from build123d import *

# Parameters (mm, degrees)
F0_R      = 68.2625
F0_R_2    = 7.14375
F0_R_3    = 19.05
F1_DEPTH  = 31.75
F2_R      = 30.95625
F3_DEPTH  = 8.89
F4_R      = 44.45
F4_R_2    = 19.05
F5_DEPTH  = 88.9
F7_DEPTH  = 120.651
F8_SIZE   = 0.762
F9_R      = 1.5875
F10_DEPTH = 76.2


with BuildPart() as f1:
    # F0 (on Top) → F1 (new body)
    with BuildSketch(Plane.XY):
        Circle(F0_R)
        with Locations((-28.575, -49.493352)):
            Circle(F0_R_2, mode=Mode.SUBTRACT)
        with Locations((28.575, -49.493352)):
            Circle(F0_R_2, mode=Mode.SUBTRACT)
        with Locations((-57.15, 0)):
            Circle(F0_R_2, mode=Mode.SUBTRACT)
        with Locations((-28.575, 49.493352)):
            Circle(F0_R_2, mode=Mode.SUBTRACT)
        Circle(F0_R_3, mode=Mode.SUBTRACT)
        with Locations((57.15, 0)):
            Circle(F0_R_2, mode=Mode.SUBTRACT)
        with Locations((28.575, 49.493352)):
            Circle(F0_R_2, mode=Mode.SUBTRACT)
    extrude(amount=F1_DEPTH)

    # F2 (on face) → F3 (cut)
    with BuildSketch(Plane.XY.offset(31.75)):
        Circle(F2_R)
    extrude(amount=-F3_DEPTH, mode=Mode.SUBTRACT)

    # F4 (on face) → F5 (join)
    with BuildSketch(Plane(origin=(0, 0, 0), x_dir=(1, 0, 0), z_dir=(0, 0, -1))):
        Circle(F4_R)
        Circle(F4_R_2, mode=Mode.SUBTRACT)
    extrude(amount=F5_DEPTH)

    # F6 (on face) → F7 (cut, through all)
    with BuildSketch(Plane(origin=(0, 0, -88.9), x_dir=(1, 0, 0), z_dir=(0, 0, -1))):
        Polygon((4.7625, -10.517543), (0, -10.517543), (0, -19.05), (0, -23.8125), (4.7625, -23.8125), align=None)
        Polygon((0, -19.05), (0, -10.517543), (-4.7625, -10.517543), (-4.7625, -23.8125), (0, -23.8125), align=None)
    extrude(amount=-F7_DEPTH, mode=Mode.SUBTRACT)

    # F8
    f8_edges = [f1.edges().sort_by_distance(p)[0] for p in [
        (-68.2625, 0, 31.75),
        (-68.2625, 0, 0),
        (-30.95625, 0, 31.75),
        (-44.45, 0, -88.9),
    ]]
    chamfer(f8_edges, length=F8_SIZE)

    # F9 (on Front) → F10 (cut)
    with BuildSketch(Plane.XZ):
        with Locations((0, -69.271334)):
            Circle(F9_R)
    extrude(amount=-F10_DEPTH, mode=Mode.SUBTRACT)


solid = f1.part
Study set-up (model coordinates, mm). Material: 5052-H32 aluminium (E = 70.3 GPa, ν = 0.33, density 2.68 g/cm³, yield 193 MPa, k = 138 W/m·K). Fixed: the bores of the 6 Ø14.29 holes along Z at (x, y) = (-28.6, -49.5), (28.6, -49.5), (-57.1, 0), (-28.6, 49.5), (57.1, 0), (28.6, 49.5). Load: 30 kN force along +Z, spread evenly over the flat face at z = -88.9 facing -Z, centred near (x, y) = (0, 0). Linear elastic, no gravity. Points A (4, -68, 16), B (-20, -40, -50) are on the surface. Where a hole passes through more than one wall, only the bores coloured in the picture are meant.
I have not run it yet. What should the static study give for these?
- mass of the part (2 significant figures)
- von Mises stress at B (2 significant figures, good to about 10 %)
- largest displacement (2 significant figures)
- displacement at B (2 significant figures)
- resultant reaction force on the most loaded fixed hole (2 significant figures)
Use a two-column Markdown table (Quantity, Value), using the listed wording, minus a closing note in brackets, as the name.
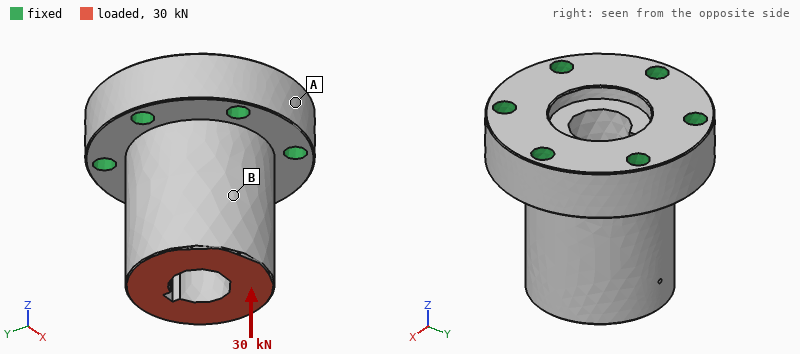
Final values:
| Quantity | Value |
|---|---|
| mass of the part | 2.2 kg |
| von Mises stress at B | 5.5 MPa |
| largest displacement | 11 µm |
| displacement at B | 7.9 µm |
| resultant reaction force on the most loaded fixed hole | 5.5 kN |
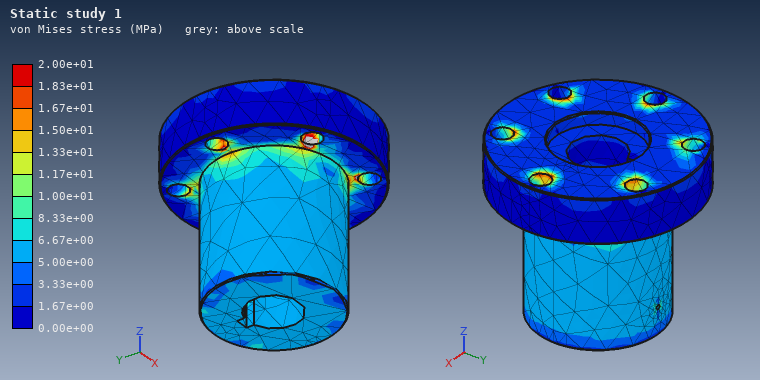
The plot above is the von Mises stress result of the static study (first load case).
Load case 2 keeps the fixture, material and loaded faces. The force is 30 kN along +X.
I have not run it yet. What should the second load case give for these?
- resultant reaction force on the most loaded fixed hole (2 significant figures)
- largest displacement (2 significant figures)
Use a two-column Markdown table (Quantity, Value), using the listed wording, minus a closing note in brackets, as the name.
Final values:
| Quantity | Value |
|---|---|
| resultant reaction force on the most loaded fixed hole | 22 kN |
| largest displacement | 0.11 mm |
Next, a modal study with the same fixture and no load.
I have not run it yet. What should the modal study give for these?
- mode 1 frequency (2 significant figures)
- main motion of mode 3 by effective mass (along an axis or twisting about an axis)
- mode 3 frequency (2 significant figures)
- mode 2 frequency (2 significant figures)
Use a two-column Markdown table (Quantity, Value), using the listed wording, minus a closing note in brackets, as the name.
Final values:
| Quantity | Value |
|---|---|
| mode 1 frequency | 4400 Hz |
| main motion of mode 3 by effective mass | twisting about Z |
| mode 3 frequency | 7900 Hz |
| mode 2 frequency | 4400 Hz |
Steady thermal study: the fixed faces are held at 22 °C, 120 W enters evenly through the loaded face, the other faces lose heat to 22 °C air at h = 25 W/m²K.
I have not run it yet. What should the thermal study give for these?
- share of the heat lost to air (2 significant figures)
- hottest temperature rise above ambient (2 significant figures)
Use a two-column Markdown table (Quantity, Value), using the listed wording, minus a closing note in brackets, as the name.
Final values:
| Quantity | Value |
|---|---|
| share of the heat lost to air | 8.4 % |
| hottest temperature rise above ambient | 18 K |
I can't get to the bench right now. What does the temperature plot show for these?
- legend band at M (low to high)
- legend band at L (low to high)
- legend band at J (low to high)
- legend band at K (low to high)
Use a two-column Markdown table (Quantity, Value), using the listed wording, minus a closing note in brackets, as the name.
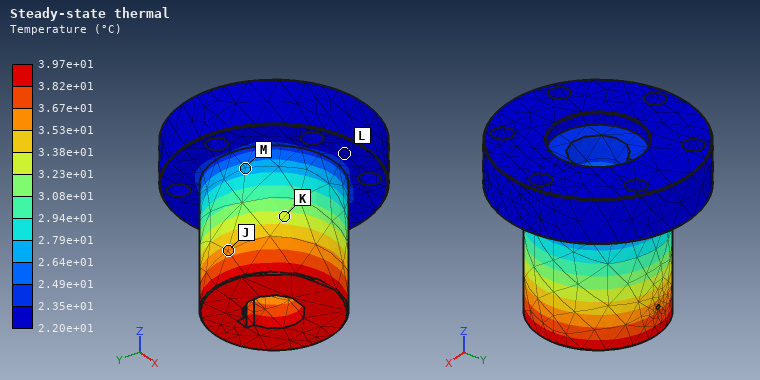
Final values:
| Quantity | Value |
|---|---|
| legend band at M | 2.64e+01 to 2.79e+01 °C |
| legend band at L | 2.20e+01 to 2.35e+01 °C |
| legend band at J | 3.53e+01 to 3.67e+01 °C |
| legend band at K | 3.23e+01 to 3.38e+01 °C |
